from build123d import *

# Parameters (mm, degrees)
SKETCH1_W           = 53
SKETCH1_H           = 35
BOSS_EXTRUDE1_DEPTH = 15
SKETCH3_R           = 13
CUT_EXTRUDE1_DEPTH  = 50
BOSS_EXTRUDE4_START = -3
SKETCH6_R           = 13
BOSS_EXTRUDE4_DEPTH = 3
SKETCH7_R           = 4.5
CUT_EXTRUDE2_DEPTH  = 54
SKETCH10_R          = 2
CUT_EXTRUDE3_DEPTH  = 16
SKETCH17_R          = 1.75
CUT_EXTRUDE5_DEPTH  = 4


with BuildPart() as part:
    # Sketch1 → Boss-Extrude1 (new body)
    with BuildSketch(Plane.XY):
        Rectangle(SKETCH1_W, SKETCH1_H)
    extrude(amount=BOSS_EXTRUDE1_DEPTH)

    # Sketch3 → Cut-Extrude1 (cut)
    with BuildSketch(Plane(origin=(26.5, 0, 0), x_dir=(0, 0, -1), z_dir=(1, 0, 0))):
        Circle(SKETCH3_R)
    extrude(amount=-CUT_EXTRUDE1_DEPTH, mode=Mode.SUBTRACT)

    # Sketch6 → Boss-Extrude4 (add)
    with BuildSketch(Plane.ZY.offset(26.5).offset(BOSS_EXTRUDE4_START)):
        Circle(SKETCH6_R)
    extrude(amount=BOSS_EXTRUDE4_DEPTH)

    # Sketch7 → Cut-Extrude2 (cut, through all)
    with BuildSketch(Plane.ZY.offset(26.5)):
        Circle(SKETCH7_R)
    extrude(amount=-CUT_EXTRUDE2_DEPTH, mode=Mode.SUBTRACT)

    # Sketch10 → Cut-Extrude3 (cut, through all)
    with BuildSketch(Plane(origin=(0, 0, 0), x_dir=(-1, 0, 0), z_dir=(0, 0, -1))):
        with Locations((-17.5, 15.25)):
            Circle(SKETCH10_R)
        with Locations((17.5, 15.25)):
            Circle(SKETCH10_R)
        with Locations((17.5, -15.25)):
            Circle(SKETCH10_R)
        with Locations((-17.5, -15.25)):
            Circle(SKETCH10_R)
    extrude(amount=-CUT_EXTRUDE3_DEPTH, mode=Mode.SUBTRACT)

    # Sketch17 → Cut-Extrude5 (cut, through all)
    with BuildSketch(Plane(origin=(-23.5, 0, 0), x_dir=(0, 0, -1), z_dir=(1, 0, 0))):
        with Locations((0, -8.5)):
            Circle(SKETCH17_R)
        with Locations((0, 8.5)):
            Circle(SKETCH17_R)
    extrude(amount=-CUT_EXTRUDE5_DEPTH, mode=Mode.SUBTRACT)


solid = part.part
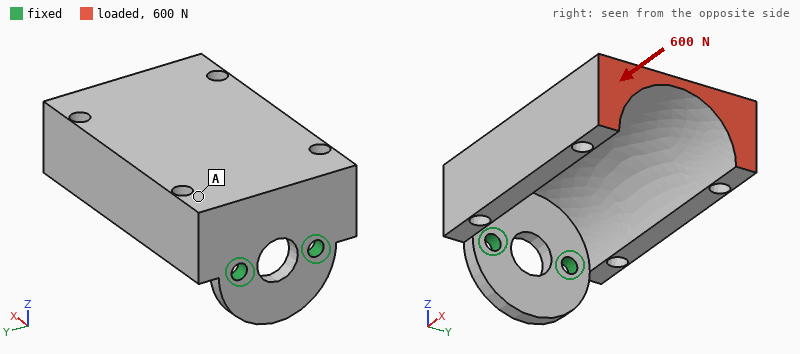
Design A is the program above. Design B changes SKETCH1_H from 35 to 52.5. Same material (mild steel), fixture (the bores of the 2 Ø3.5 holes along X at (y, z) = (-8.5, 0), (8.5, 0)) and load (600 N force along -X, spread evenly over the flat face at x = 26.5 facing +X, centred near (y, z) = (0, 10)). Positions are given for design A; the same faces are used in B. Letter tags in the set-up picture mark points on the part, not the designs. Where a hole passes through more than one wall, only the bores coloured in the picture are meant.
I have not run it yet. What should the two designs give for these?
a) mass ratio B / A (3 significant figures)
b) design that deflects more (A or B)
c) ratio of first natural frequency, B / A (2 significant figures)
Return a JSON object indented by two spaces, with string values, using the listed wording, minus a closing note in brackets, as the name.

{
  "mass ratio B / A": "1.97",
  "design that deflects more": "A",
  "ratio of first natural frequency, B / A": "0.72"
}
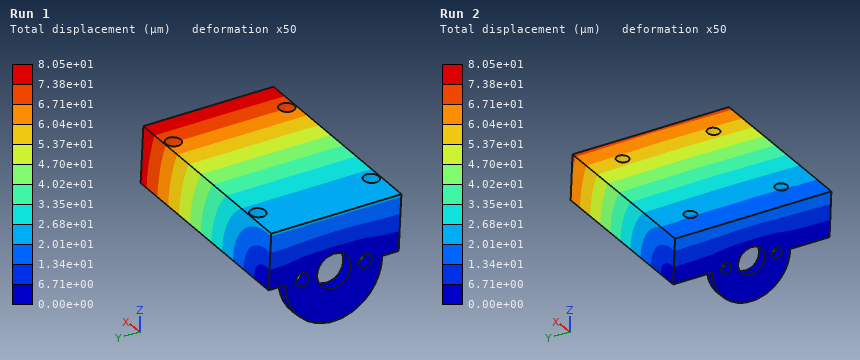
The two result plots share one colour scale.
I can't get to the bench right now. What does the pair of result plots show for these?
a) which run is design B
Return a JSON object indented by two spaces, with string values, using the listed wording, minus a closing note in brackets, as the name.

{
  "which run is design B": "Run 2"
}
